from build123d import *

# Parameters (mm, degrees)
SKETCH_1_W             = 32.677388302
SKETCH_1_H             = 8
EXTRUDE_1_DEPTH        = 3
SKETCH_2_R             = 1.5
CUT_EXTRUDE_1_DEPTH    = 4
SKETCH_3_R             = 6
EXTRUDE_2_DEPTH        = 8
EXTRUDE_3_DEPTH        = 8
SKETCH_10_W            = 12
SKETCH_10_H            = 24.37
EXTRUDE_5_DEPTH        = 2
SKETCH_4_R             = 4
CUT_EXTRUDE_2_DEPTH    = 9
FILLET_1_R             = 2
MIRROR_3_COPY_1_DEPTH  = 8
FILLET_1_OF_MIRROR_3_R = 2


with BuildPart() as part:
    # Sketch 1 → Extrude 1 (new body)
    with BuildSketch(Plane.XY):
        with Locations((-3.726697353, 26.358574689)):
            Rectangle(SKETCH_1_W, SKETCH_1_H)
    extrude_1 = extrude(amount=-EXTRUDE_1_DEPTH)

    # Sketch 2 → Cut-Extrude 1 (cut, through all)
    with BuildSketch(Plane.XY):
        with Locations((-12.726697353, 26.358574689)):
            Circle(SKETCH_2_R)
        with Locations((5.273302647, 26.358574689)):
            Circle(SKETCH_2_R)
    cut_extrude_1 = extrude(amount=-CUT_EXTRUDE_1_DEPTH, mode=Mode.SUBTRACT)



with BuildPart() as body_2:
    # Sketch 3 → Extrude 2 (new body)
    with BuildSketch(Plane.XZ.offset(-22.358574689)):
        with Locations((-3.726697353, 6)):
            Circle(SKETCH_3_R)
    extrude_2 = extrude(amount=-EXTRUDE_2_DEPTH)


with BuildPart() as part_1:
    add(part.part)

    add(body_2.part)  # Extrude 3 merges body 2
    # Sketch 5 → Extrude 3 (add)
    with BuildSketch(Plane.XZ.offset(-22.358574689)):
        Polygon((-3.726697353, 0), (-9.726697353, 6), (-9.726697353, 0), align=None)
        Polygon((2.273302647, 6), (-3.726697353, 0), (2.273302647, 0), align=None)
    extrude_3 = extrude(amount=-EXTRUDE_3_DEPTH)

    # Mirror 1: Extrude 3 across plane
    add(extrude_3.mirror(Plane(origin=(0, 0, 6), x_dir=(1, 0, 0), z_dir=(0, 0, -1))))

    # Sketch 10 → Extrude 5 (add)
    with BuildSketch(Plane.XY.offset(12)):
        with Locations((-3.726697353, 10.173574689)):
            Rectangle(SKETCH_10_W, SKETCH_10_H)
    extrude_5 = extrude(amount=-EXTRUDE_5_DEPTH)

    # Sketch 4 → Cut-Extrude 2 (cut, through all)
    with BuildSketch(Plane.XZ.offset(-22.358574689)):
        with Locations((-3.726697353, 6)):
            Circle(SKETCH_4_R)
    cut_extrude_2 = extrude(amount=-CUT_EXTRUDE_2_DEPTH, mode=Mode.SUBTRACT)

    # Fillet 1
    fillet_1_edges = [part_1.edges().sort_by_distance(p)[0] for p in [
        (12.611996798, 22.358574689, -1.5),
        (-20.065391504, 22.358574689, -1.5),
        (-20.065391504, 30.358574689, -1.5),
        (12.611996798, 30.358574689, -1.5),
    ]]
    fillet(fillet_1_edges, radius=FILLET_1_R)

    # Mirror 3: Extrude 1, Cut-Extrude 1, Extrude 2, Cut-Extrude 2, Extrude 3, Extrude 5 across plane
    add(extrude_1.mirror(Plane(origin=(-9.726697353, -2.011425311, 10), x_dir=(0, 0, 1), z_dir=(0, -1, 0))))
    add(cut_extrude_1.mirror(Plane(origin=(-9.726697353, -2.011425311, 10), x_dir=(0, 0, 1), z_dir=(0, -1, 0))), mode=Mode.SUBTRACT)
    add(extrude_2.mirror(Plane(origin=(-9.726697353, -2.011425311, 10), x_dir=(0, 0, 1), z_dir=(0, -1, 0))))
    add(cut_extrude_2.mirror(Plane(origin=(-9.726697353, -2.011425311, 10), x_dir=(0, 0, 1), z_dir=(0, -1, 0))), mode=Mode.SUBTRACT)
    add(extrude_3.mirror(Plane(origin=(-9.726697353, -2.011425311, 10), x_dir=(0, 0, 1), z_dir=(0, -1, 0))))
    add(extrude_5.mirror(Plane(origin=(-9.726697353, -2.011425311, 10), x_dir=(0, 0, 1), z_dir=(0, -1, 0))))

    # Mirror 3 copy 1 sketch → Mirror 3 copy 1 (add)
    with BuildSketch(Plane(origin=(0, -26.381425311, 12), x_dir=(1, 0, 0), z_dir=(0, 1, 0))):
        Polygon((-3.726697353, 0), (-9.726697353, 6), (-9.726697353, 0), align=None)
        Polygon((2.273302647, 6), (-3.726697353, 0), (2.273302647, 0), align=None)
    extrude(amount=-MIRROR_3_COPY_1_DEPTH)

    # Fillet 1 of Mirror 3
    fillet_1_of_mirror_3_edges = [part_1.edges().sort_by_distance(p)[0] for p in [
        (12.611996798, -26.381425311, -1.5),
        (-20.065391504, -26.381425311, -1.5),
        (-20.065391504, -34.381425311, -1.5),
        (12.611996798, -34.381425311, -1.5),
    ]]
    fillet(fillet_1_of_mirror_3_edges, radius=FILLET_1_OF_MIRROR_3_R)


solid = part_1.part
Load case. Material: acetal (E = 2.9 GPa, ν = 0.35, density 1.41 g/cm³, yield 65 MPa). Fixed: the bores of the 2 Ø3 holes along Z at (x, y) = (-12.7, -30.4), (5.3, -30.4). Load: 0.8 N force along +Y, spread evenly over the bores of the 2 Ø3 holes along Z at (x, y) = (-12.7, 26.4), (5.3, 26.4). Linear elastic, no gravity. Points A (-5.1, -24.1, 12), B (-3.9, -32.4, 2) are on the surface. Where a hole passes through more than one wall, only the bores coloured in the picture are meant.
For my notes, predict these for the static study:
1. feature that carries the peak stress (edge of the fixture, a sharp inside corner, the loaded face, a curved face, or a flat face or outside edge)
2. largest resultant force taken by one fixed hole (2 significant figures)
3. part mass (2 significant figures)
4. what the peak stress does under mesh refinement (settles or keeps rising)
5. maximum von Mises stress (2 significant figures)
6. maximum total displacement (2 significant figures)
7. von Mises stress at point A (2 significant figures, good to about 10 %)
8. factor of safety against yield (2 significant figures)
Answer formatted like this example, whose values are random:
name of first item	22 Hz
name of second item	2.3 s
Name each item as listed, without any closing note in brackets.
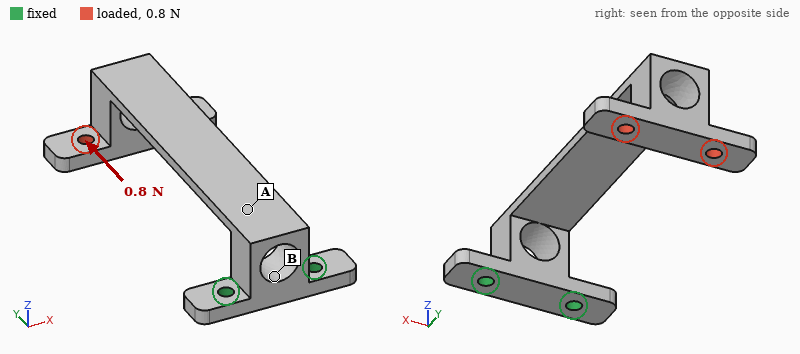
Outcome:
feature that carries the peak stress	a flat face or outside edge
largest resultant force taken by one fixed hole	0.40 N
part mass	5.8 g
what the peak stress does under mesh refinement	settles
maximum von Mises stress	1.3 MPa
maximum total displacement	0.78 mm
von Mises stress at point A	1.1 MPa
factor of safety against yield	50
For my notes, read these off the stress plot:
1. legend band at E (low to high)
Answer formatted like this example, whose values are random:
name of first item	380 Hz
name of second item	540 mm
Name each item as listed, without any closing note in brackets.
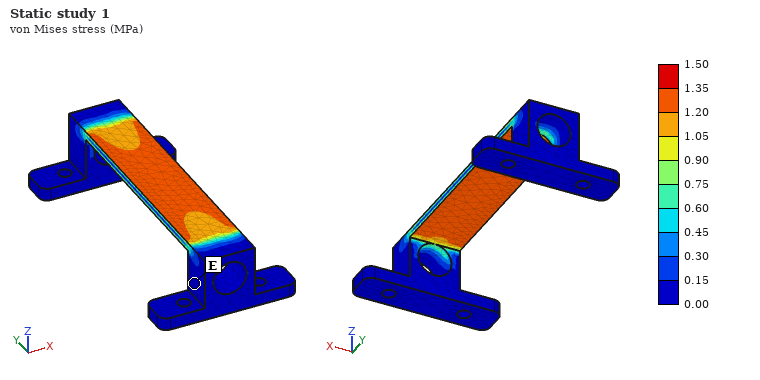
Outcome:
legend band at E	0.00 to 0.15 MPa
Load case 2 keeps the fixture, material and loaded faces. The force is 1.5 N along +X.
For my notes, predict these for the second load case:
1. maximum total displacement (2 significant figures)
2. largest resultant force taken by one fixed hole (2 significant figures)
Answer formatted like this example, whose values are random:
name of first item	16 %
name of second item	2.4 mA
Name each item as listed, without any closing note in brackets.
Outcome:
maximum total displacement	0.83 mm
largest resultant force taken by one fixed hole	5.0 N
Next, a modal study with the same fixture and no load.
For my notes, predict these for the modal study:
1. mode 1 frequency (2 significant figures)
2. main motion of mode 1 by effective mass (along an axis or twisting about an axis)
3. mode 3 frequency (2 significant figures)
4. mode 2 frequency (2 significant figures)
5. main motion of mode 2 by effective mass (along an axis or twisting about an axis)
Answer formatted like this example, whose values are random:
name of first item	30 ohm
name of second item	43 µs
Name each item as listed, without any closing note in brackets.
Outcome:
mode 1 frequency	65 Hz
main motion of mode 1 by effective mass	along Z
mode 3 frequency	390 Hz
mode 2 frequency	180 Hz
main motion of mode 2 by effective mass	along X
